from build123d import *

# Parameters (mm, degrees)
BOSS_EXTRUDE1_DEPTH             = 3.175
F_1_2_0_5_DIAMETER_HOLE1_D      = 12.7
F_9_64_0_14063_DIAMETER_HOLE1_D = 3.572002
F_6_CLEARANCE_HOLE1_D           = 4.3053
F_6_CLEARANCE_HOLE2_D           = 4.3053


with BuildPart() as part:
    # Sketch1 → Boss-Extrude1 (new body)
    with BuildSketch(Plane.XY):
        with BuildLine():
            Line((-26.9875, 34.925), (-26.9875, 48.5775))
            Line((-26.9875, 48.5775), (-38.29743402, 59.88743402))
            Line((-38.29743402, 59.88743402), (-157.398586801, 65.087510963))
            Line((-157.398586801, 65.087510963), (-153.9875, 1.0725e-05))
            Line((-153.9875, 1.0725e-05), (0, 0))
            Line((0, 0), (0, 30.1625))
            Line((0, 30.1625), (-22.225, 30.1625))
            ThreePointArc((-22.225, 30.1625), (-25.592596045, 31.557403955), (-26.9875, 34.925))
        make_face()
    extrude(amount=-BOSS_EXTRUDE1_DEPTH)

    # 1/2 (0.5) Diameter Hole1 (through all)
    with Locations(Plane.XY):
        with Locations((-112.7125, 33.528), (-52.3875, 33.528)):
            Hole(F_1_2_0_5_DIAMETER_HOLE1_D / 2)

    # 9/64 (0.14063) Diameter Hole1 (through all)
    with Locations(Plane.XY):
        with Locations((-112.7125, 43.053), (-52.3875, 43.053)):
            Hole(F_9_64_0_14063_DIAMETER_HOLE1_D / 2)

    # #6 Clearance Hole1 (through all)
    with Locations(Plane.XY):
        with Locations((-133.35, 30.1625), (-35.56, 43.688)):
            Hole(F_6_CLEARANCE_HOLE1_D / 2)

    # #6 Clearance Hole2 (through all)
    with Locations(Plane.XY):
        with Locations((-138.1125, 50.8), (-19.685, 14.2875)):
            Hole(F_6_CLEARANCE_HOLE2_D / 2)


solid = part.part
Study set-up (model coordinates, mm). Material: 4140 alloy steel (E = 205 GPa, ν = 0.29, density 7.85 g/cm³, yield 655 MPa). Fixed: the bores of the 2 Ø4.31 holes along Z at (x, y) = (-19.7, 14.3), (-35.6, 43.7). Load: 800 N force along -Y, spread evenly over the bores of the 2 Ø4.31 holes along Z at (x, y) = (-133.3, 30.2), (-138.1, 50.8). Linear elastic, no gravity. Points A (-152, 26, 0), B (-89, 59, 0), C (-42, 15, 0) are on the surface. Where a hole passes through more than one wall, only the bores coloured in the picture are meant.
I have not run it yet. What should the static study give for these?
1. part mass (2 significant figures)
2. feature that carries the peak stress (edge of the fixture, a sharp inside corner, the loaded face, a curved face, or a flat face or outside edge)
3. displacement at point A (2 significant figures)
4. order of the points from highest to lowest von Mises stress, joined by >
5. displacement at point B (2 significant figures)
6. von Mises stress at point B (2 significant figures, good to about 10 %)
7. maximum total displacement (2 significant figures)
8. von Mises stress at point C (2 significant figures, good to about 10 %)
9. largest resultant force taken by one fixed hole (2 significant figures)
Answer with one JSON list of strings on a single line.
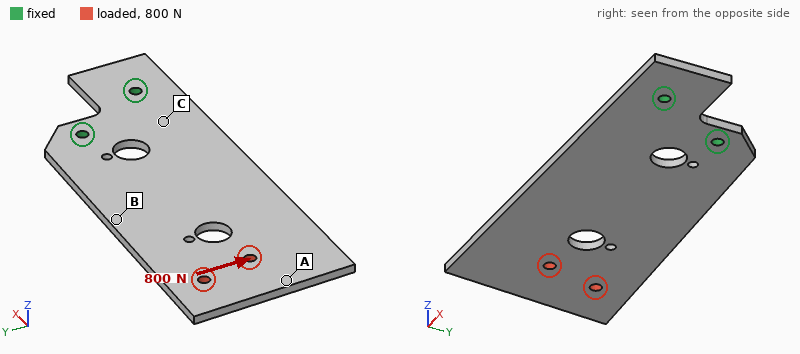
["210 g", "edge of the fixture", "62 µm", "C > B > A", "29 µm", "17 MPa", "68 µm", "28 MPa", "2.6 kN"]
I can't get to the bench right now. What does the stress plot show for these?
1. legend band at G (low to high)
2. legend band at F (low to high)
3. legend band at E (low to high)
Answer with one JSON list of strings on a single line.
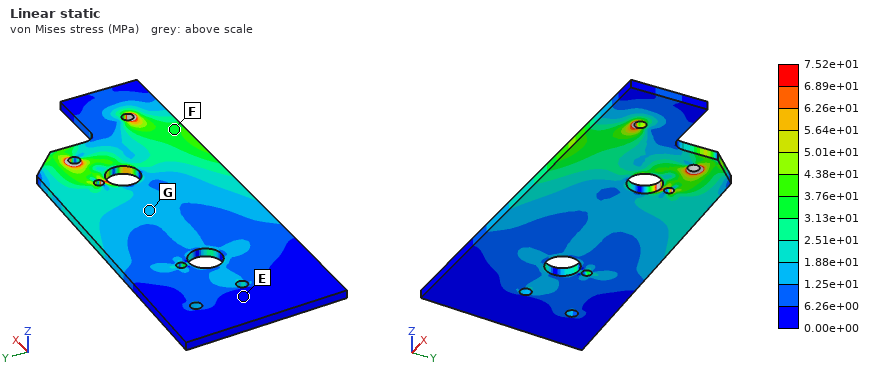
["1.25e+01 to 1.88e+01 MPa", "3.13e+01 to 3.76e+01 MPa", "0.00e+00 to 6.26e+00 MPa"]
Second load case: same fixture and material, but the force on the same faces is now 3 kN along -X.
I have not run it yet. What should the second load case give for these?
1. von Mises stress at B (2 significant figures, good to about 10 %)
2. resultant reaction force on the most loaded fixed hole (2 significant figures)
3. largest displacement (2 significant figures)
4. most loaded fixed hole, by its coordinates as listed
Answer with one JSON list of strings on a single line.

["31 MPa", "2.5 kN", "33 µm", "(-35.6, 43.7)"]
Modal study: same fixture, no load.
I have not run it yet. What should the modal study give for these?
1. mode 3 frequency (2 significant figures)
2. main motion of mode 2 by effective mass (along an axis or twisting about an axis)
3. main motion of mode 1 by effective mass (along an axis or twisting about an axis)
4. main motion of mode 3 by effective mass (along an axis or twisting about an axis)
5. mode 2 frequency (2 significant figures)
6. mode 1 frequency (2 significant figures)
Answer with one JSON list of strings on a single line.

["1000 Hz", "twisting about X", "along Z", "along Z", "630 Hz", "160 Hz"]
